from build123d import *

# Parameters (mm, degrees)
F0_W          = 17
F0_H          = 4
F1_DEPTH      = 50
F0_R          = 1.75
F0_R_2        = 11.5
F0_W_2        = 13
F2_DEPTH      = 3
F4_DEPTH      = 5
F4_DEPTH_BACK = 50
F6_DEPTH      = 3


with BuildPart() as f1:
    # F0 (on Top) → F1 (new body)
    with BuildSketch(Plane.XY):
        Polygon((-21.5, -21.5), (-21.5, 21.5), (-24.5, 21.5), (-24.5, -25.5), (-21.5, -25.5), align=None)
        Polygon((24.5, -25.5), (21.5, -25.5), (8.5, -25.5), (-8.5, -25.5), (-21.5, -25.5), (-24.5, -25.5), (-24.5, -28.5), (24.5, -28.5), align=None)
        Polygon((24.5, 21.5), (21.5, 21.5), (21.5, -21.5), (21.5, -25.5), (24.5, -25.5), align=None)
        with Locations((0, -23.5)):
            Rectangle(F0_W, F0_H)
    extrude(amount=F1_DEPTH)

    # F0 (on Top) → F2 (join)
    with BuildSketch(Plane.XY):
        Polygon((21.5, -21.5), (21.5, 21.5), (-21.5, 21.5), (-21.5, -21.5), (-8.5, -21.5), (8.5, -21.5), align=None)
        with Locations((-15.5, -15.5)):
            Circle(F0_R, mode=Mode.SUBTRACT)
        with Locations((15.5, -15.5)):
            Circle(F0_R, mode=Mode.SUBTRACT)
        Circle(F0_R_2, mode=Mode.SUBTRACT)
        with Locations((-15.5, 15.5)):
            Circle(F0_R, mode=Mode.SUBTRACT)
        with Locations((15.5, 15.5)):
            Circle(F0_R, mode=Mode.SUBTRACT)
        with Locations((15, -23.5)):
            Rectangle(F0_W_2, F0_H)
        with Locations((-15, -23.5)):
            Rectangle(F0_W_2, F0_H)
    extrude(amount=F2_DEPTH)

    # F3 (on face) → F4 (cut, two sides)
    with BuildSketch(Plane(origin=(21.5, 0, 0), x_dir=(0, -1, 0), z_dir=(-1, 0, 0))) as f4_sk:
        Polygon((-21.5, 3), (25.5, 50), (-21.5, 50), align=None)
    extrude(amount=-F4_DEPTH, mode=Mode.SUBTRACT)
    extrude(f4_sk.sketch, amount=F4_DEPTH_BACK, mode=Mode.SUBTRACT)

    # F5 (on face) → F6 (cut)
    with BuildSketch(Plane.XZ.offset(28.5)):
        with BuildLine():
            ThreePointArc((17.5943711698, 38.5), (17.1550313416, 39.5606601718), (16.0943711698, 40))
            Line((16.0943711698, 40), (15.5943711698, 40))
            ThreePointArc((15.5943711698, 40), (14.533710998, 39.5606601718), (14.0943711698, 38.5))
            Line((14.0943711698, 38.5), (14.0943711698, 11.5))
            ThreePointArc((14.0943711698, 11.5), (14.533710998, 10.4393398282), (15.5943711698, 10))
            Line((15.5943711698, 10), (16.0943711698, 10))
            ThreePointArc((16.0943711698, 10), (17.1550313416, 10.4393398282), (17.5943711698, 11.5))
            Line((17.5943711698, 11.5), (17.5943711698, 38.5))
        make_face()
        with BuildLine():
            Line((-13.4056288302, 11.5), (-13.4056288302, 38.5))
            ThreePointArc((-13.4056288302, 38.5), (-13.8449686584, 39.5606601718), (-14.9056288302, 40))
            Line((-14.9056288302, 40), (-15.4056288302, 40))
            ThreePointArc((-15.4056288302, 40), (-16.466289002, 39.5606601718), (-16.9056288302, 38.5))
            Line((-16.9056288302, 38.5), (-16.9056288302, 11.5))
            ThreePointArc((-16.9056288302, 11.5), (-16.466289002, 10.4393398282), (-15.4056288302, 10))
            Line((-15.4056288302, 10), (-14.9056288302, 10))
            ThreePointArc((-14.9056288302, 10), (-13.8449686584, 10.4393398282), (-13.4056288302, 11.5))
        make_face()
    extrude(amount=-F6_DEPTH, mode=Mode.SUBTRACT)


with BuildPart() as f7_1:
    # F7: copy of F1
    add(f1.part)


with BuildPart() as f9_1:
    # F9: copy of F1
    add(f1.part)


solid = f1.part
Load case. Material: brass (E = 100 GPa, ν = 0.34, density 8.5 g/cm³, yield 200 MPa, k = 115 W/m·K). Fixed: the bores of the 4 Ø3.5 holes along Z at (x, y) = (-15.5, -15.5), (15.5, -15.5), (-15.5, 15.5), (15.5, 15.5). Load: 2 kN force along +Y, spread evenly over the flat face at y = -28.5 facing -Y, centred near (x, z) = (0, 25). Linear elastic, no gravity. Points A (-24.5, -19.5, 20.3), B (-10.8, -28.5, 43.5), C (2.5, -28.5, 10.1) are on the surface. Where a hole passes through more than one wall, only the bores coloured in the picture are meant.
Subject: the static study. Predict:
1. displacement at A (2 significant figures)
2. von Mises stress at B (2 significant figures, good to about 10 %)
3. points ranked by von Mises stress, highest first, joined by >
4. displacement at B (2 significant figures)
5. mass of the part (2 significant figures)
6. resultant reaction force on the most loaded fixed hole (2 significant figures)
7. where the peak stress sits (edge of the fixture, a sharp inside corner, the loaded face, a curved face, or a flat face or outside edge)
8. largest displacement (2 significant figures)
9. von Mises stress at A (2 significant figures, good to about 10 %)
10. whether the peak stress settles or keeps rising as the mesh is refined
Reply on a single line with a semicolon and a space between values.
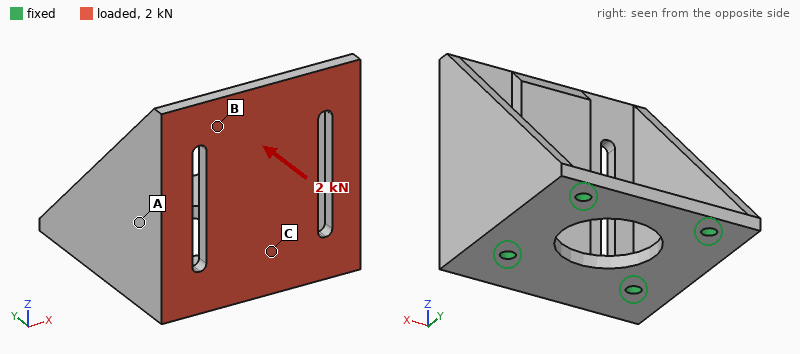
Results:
0.034 mm; 110 MPa; B > A > C; 0.16 mm; 190 g; 970 N; edge of the fixture; 0.19 mm; 32 MPa; keeps rising
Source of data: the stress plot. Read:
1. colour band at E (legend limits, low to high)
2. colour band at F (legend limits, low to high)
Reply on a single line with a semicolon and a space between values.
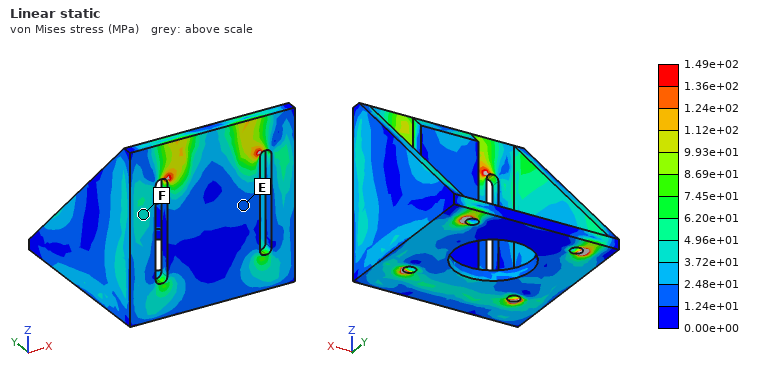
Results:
1.24e+01 to 2.48e+01 MPa; 3.72e+01 to 4.96e+01 MPa
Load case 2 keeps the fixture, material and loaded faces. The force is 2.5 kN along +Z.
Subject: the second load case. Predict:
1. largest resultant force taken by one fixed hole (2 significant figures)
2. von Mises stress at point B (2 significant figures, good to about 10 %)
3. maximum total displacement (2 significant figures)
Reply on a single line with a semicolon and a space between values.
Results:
1.7 kN; 27 MPa; 0.10 mm
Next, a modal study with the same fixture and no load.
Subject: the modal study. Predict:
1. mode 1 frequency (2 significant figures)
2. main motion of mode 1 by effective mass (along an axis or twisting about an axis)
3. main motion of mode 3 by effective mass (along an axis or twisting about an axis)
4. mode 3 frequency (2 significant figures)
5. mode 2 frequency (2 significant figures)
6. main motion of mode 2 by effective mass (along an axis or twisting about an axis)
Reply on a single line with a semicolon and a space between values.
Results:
2000 Hz; along Y; along Z; 3600 Hz; 2100 Hz; along X
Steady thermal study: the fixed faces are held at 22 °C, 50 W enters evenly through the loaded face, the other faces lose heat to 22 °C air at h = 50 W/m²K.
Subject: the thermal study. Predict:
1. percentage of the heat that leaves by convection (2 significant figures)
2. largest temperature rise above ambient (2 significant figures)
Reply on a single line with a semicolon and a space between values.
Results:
23 %; 48 K
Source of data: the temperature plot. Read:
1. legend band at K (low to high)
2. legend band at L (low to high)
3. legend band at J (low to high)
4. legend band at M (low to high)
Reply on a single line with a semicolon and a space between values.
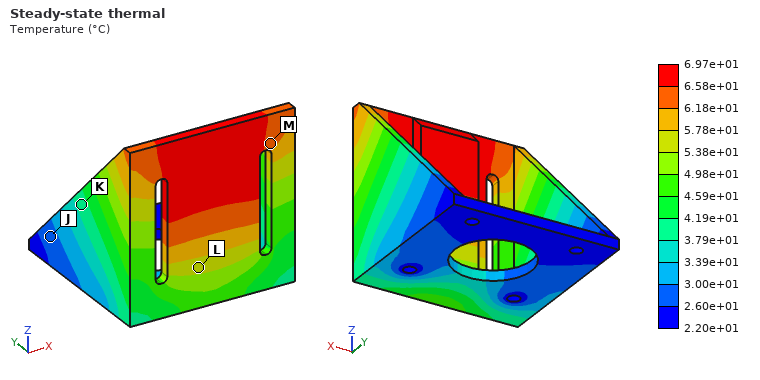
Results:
3.79e+01 to 4.19e+01 °C; 5.38e+01 to 5.78e+01 °C; 2.60e+01 to 3.00e+01 °C; 6.18e+01 to 6.58e+01 °C
